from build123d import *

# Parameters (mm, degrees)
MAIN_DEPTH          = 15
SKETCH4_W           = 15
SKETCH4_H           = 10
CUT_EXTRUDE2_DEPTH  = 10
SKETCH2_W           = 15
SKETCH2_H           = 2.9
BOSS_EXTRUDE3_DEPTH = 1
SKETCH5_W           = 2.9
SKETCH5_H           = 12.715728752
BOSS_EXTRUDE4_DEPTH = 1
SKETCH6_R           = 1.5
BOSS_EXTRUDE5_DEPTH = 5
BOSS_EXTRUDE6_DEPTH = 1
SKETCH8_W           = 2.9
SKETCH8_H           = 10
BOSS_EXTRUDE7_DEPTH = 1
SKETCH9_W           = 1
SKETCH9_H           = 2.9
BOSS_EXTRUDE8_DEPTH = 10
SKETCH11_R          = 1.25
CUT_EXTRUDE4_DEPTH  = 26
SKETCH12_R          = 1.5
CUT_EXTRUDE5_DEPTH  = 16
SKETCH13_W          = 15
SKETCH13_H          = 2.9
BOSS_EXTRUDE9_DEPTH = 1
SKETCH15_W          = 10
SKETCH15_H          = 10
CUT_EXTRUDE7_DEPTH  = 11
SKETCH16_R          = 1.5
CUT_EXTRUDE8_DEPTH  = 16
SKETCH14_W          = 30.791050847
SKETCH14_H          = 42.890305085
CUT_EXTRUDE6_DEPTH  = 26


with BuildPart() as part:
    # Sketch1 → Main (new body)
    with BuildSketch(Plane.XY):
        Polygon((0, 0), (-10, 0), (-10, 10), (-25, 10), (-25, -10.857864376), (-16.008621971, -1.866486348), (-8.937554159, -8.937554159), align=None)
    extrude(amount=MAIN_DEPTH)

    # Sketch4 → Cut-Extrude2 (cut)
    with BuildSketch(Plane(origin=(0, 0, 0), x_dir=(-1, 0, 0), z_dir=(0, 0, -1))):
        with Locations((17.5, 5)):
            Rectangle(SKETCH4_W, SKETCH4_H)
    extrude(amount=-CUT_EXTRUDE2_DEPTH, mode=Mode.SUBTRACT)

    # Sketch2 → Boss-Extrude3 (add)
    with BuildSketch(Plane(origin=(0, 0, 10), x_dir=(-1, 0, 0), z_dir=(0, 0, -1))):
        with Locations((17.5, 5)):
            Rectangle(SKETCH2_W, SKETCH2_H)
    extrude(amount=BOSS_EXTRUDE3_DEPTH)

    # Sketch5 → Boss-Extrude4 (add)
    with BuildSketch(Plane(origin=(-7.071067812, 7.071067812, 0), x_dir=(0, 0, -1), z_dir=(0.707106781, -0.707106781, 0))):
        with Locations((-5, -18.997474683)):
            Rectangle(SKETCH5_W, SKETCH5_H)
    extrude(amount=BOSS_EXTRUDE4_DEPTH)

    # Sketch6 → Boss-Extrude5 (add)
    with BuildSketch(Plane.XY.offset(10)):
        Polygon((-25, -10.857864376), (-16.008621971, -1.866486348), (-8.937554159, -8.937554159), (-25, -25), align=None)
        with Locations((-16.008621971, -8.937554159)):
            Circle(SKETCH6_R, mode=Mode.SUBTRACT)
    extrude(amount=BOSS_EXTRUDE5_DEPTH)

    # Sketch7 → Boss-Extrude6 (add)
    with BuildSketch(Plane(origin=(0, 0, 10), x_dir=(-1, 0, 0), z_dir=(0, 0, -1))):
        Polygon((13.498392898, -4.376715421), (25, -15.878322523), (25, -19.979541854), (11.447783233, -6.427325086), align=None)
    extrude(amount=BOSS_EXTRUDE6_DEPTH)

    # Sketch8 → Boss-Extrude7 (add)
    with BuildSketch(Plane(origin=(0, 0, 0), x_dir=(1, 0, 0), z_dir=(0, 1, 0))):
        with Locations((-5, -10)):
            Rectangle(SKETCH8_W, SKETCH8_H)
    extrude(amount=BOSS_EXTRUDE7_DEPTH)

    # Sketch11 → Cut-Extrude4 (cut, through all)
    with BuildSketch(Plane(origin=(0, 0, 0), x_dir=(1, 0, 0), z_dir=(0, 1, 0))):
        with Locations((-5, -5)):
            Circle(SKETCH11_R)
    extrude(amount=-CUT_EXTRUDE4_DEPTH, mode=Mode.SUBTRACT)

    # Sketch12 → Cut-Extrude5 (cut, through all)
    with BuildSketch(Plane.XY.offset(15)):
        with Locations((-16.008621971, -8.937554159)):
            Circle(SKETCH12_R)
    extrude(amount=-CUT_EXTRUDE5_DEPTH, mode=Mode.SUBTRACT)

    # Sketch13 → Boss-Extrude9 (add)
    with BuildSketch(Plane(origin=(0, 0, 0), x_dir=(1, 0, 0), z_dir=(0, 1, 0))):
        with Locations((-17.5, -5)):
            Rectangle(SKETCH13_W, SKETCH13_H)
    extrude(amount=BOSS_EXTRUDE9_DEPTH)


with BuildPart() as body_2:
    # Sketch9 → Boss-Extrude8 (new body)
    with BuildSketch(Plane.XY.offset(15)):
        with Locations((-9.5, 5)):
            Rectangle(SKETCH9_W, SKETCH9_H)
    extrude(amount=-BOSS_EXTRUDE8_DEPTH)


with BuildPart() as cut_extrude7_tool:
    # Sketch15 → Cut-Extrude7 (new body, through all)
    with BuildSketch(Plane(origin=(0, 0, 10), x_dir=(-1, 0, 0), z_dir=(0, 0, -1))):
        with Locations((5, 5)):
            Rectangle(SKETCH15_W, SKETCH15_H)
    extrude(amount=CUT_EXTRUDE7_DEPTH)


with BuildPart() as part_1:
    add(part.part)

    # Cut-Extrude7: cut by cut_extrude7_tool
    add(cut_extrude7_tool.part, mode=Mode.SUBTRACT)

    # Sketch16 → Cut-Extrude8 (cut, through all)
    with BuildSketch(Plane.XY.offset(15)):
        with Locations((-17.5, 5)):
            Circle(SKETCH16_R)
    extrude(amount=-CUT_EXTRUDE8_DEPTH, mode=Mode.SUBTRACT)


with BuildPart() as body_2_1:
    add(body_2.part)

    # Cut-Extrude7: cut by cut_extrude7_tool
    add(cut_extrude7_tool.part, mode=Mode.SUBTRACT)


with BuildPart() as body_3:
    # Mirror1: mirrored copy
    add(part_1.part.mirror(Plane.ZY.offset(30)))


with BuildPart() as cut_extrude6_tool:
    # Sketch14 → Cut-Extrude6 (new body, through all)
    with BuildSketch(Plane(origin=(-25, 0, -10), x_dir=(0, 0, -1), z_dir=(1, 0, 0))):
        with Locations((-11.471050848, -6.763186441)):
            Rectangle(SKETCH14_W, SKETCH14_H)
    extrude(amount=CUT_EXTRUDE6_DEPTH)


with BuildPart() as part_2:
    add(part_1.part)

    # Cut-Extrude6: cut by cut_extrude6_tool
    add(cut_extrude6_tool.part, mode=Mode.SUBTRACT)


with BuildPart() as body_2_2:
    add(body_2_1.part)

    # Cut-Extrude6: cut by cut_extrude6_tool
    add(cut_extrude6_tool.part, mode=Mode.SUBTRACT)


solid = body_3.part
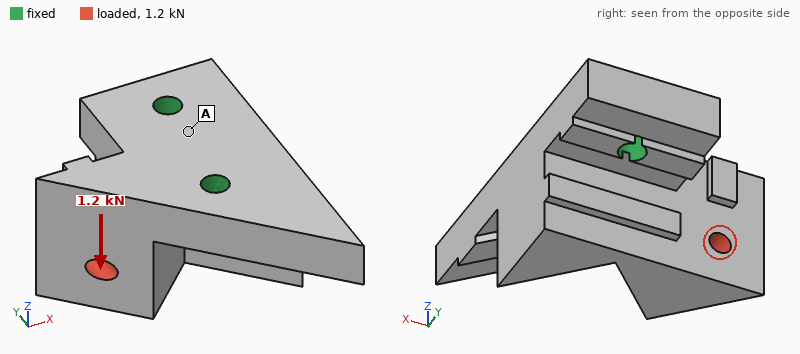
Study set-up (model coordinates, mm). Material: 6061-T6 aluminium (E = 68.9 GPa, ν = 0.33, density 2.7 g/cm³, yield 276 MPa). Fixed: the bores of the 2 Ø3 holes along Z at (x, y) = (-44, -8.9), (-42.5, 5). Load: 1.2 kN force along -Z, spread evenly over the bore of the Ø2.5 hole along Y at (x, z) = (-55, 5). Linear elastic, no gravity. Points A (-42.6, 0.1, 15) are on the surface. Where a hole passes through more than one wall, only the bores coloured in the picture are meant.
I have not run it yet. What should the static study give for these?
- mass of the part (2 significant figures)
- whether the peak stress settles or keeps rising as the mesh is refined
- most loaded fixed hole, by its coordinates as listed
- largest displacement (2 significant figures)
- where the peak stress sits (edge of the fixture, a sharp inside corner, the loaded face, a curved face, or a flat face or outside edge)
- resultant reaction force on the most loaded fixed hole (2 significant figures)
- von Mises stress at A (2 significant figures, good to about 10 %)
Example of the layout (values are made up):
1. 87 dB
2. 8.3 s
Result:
1. 10 g
2. keeps rising
3. (-44, -8.9)
4. 68 µm
5. edge of the fixture
6. 820 N
7. 32 MPa
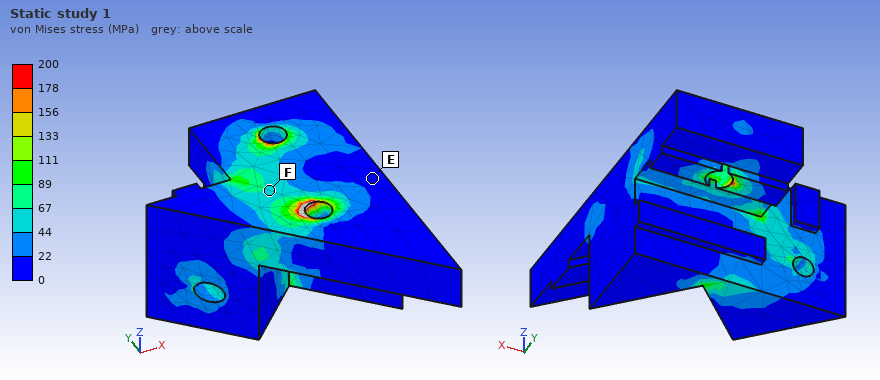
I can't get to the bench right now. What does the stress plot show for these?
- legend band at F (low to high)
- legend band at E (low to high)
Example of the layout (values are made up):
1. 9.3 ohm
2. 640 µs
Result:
1. 44 to 67 MPa
2. 0 to 22 MPa
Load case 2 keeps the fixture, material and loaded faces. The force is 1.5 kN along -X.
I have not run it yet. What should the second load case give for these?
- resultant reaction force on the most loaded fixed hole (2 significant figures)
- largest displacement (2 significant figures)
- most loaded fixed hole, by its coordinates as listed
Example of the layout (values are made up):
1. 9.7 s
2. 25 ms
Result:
1. 850 N
2. 52 µm
3. (-44, -8.9)
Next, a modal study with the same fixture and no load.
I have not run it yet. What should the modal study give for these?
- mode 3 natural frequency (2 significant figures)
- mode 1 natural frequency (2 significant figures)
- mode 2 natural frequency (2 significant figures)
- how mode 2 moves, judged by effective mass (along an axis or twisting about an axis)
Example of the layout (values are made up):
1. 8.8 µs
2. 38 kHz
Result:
1. 24 kHz
2. 15 kHz
3. 23 kHz
4. along Y
